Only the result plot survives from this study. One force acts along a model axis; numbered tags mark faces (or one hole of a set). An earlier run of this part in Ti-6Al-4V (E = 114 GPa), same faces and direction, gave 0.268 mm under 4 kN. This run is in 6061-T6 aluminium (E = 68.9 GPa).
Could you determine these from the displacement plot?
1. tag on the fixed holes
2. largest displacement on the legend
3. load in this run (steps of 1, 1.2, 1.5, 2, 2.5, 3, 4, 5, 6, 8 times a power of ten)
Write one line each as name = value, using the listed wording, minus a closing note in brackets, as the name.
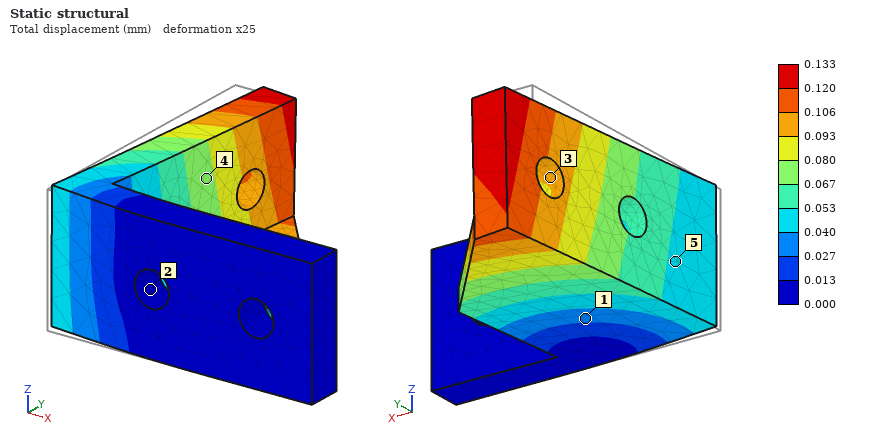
tag on the fixed holes = 2
largest displacement on the legend = 0.133 mm
load in this run = 1.2 kN
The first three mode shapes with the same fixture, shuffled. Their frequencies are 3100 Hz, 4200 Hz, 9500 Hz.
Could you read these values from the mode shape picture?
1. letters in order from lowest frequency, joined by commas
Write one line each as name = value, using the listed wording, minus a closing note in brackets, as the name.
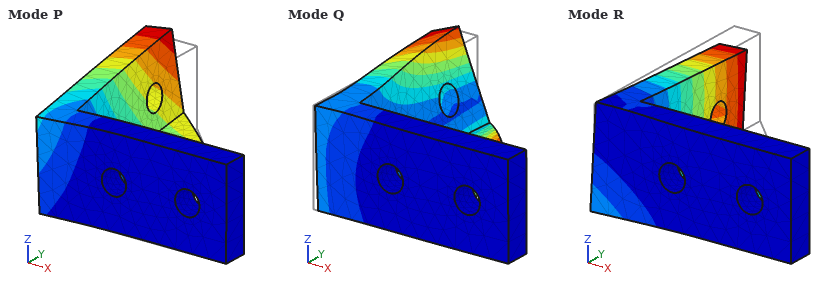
letters in order from lowest frequency, joined by commas = R, P, Q
